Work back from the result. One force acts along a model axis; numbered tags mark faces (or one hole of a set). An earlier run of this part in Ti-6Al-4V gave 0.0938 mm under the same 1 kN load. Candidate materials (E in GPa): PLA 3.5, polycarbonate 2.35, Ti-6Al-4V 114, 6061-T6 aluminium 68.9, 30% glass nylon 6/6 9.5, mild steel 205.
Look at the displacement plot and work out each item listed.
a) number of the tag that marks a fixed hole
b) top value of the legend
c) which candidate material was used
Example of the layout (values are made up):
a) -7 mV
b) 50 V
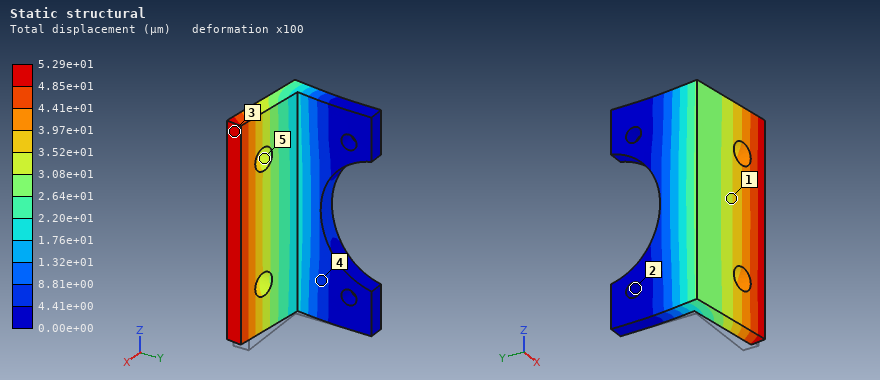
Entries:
a) 2
b) 5.29e+01 µm
c) mild steel
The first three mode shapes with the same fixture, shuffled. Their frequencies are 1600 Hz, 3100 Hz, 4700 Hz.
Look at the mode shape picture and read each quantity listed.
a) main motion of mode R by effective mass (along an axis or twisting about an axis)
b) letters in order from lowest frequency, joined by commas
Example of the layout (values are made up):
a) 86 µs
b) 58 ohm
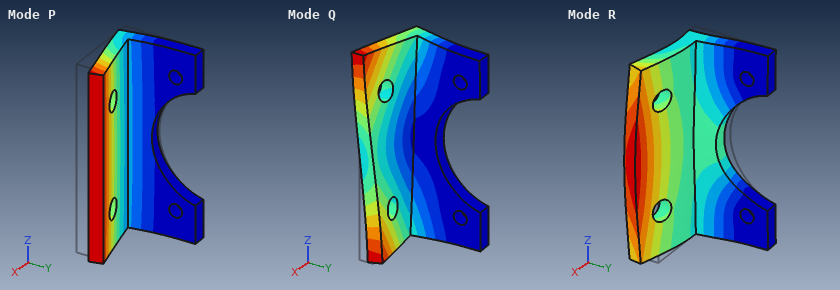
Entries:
a) along X
b) P, Q, R
